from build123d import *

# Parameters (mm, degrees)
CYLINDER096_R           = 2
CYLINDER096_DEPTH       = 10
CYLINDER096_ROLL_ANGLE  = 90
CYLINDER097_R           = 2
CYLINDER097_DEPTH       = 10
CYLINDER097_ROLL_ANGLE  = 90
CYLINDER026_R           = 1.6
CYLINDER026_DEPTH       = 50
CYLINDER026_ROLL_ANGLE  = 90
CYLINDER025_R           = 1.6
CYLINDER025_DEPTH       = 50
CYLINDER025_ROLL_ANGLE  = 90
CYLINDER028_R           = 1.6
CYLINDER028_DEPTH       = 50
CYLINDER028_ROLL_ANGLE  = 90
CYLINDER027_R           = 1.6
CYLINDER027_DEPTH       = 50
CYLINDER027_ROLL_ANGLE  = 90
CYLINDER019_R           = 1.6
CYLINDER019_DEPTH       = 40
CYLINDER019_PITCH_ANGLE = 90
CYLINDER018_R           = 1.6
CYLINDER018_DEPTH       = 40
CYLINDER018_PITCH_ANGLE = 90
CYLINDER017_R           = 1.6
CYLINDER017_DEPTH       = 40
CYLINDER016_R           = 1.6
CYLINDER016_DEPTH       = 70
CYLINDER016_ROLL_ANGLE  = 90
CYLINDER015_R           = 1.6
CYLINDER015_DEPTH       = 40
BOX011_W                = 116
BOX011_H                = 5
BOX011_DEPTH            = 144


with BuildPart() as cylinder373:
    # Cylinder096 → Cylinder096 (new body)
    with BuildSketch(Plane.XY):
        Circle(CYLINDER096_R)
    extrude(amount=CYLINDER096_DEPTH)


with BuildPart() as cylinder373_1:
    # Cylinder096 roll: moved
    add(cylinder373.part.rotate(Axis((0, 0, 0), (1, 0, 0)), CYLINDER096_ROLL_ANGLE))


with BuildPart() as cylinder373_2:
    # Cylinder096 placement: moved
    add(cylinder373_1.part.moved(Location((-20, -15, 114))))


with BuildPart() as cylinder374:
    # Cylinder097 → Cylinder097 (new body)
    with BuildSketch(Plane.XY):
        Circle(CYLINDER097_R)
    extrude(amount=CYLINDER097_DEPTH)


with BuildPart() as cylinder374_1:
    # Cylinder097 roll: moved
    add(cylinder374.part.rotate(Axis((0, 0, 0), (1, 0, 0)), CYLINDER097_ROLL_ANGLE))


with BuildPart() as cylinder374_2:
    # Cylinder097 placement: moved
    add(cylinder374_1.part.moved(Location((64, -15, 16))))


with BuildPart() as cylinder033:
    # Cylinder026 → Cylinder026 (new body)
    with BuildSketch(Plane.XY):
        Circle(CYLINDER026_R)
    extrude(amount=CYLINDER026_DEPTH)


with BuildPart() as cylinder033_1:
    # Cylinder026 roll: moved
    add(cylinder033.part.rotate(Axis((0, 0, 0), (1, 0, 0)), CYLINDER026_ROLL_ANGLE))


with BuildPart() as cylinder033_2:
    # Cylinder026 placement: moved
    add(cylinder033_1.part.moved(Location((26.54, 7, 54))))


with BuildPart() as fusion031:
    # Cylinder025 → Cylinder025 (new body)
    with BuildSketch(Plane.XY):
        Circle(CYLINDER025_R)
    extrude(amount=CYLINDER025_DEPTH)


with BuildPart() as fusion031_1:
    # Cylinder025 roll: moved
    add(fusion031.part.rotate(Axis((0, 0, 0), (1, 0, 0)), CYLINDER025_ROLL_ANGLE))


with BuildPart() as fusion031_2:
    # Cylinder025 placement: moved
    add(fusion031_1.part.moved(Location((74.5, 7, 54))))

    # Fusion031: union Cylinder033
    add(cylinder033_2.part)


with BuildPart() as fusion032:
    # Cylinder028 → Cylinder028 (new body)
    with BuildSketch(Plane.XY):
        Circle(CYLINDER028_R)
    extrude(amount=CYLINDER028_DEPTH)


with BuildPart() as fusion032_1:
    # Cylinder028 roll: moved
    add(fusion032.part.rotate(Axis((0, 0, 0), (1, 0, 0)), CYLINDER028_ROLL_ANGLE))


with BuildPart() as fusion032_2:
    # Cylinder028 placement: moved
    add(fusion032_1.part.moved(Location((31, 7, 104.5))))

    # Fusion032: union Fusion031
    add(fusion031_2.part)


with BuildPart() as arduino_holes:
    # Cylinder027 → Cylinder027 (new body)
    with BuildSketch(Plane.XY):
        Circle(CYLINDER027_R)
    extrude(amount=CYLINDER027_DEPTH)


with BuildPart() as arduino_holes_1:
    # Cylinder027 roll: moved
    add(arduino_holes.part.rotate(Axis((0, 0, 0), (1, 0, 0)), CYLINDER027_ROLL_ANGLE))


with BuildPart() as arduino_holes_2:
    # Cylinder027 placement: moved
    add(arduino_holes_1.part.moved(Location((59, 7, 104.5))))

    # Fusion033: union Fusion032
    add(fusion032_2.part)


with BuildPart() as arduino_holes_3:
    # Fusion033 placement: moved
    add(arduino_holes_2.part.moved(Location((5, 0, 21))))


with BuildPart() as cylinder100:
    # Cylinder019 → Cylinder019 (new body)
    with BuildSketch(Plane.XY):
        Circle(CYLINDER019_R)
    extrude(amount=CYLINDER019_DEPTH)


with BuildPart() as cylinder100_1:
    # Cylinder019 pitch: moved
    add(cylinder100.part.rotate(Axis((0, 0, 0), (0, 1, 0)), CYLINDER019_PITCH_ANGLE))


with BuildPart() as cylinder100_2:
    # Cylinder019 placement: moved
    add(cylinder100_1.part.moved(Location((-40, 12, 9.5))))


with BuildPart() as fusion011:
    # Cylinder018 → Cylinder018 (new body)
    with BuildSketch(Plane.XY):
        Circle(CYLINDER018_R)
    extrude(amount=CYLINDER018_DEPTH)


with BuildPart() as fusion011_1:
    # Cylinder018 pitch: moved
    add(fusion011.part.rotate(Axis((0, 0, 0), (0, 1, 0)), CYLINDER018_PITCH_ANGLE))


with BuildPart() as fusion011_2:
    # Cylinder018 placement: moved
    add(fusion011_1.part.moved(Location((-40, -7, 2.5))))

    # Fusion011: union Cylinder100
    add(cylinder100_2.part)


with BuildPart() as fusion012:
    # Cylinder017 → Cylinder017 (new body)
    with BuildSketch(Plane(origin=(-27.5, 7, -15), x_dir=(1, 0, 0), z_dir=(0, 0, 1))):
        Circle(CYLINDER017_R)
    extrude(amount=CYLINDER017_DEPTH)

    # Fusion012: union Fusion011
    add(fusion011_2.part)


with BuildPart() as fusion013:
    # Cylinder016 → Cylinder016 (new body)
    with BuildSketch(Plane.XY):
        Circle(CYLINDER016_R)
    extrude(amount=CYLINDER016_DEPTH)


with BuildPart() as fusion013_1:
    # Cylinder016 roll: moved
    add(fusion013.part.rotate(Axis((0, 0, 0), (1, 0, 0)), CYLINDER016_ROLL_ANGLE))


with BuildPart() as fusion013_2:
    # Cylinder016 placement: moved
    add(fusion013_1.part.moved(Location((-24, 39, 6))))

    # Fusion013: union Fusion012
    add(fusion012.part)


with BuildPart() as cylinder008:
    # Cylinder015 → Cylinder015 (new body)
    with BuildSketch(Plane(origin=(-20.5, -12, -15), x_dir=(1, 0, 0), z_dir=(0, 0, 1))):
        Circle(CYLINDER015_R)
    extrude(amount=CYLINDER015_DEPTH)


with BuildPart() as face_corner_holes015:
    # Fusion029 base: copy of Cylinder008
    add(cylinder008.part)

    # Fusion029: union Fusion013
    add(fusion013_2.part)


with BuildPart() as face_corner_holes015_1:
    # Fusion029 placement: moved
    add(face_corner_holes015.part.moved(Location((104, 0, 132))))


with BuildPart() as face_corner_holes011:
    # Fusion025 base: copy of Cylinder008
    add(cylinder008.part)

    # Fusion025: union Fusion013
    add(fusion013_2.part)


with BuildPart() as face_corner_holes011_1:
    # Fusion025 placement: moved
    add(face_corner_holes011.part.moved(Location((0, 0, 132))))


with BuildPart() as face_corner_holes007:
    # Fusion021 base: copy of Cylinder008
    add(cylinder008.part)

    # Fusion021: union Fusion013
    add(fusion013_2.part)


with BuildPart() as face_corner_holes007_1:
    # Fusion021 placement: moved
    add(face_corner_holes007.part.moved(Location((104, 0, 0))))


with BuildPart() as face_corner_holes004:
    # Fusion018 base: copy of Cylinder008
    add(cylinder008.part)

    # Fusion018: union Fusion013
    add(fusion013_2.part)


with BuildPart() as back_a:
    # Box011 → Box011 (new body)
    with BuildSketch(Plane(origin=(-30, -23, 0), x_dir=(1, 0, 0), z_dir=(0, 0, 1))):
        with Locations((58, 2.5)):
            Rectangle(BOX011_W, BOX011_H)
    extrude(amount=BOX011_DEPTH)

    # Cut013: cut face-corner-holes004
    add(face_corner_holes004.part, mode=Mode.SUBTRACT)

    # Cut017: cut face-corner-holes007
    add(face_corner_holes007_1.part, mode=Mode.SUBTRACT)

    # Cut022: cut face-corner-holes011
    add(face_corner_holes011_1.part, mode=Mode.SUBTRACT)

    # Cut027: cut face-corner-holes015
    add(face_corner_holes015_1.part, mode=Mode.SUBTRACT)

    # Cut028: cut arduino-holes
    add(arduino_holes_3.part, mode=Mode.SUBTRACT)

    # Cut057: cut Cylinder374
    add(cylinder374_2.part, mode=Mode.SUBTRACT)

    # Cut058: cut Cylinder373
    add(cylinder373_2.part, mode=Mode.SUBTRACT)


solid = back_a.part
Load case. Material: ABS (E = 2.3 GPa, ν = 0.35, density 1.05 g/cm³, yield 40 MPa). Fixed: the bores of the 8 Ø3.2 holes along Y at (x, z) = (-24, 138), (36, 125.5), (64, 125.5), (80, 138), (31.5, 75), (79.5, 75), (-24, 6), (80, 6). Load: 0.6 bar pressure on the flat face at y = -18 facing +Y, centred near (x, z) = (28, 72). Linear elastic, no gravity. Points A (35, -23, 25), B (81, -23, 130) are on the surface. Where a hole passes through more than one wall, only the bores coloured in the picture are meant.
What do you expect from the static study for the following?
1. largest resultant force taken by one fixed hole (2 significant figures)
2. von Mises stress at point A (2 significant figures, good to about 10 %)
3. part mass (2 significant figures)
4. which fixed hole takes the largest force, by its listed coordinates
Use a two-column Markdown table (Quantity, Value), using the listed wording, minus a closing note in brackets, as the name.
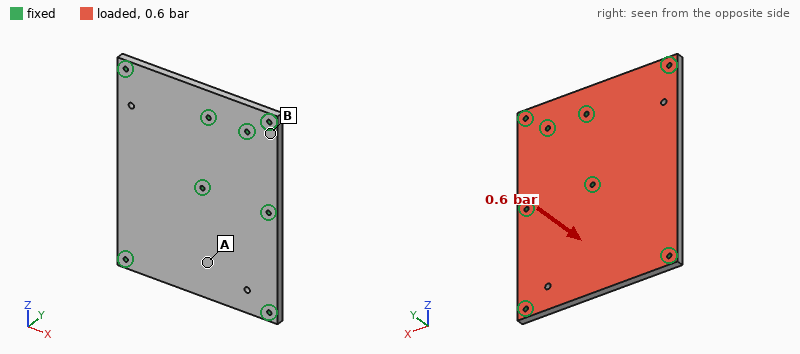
| Quantity | Value |
|---|---|
| largest resultant force taken by one fixed hole | 340 N |
| von Mises stress at point A | 3.8 MPa |
| part mass | 87 g |
| which fixed hole takes the largest force, by its listed coordinates | (31.5, 75) |
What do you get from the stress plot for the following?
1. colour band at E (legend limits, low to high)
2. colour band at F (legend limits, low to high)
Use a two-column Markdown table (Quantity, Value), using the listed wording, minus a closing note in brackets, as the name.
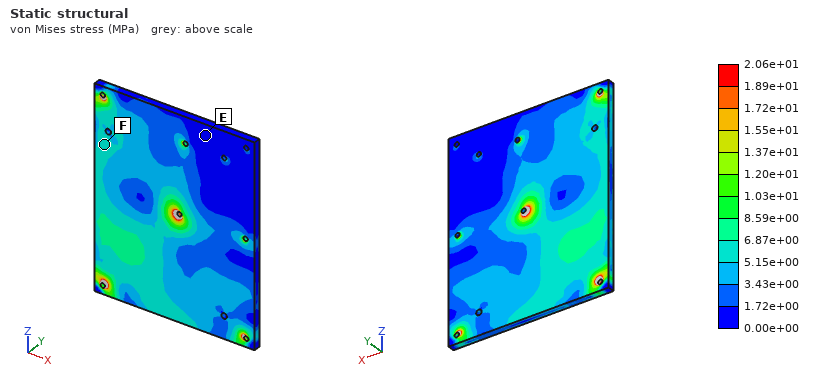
| Quantity | Value |
|---|---|
| colour band at E | 0.00e+00 to 1.72e+00 MPa |
| colour band at F | 5.15e+00 to 6.87e+00 MPa |
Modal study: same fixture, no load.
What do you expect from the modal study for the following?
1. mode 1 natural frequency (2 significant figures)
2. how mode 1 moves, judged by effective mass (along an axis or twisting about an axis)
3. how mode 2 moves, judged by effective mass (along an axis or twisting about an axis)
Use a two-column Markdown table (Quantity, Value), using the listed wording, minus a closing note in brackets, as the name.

| Quantity | Value |
|---|---|
| mode 1 natural frequency | 570 Hz |
| how mode 1 moves, judged by effective mass | along Y |
| how mode 2 moves, judged by effective mass | along Y |
